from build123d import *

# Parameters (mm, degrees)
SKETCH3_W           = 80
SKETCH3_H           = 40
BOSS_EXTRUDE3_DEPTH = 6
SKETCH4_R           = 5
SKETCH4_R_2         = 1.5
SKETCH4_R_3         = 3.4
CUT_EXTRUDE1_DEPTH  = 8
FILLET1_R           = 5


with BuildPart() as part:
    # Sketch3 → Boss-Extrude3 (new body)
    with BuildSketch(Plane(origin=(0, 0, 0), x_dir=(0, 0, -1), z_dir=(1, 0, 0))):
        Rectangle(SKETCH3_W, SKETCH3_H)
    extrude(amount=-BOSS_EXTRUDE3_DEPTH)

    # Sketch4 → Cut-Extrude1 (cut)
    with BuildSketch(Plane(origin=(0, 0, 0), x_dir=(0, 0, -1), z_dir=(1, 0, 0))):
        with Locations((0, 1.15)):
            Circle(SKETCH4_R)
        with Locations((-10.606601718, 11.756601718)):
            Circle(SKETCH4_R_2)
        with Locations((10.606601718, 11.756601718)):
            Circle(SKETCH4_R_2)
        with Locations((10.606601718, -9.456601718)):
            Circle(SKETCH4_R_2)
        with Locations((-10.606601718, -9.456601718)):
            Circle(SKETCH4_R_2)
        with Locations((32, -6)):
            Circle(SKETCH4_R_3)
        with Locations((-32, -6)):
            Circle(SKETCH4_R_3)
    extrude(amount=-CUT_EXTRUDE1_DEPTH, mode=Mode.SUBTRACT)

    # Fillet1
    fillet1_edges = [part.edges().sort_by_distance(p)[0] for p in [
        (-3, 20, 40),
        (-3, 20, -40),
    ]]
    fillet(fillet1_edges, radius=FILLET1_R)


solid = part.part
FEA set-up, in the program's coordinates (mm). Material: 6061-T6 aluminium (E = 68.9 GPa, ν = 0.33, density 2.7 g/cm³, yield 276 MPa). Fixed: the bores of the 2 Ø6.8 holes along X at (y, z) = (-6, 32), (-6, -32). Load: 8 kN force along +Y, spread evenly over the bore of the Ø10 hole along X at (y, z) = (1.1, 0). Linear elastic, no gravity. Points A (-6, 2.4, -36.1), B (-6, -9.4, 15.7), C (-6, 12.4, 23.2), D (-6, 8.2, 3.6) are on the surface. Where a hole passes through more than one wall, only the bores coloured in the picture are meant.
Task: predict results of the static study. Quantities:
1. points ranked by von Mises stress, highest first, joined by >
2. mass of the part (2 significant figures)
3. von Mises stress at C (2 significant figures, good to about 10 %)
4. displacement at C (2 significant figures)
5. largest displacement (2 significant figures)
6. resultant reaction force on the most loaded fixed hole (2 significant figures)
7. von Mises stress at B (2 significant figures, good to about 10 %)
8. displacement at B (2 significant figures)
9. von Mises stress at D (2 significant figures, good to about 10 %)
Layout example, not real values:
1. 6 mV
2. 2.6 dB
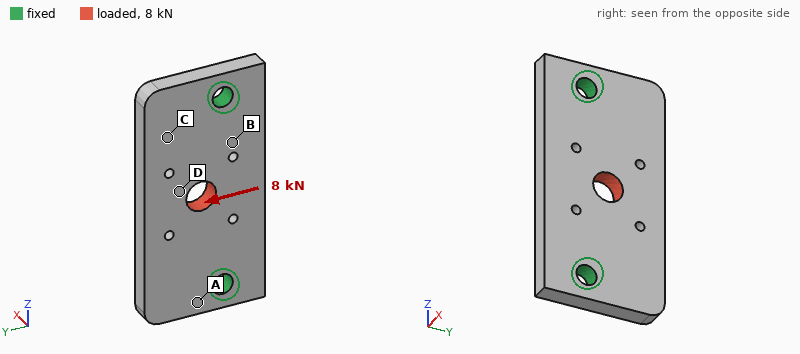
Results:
1. D > B > C > A
2. 49 g
3. 24 MPa
4. 16 µm
5. 40 µm
6. 4.2 kN
7. 40 MPa
8. 23 µm
9. 53 MPa
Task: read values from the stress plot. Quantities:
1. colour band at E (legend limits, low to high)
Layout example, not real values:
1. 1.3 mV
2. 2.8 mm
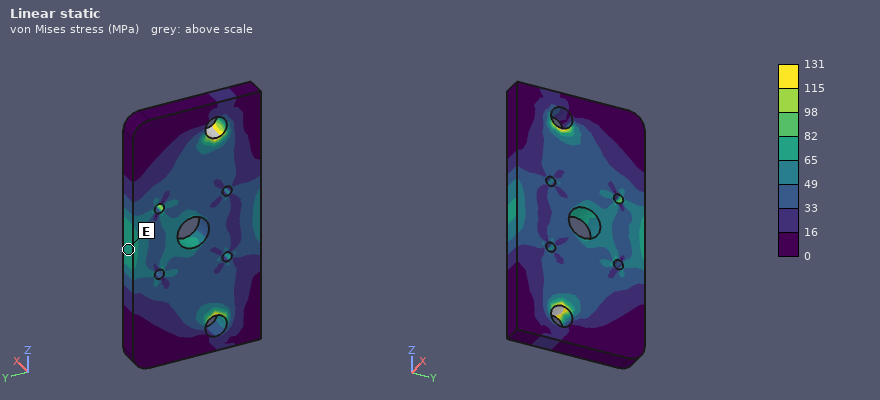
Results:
1. 65 to 82 MPa
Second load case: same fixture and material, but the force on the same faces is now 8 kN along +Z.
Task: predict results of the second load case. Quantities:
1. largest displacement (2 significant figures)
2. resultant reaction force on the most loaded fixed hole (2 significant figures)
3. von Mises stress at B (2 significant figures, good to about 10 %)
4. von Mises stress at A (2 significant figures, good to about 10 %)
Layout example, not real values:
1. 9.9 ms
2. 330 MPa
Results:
1. 18 µm
2. 4.1 kN
3. 22 MPa
4. 14 MPa
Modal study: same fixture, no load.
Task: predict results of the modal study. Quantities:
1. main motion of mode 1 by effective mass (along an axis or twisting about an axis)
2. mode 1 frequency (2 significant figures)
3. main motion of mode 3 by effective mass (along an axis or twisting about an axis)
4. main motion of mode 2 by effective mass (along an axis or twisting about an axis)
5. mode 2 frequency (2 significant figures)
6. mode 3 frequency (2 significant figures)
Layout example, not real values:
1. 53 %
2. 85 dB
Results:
1. along X
2. 5000 Hz
3. twisting about Y
4. along X
5. 7900 Hz
6. 9000 Hz
